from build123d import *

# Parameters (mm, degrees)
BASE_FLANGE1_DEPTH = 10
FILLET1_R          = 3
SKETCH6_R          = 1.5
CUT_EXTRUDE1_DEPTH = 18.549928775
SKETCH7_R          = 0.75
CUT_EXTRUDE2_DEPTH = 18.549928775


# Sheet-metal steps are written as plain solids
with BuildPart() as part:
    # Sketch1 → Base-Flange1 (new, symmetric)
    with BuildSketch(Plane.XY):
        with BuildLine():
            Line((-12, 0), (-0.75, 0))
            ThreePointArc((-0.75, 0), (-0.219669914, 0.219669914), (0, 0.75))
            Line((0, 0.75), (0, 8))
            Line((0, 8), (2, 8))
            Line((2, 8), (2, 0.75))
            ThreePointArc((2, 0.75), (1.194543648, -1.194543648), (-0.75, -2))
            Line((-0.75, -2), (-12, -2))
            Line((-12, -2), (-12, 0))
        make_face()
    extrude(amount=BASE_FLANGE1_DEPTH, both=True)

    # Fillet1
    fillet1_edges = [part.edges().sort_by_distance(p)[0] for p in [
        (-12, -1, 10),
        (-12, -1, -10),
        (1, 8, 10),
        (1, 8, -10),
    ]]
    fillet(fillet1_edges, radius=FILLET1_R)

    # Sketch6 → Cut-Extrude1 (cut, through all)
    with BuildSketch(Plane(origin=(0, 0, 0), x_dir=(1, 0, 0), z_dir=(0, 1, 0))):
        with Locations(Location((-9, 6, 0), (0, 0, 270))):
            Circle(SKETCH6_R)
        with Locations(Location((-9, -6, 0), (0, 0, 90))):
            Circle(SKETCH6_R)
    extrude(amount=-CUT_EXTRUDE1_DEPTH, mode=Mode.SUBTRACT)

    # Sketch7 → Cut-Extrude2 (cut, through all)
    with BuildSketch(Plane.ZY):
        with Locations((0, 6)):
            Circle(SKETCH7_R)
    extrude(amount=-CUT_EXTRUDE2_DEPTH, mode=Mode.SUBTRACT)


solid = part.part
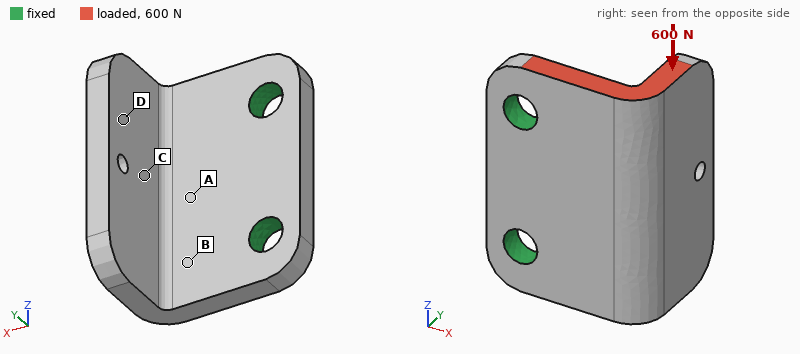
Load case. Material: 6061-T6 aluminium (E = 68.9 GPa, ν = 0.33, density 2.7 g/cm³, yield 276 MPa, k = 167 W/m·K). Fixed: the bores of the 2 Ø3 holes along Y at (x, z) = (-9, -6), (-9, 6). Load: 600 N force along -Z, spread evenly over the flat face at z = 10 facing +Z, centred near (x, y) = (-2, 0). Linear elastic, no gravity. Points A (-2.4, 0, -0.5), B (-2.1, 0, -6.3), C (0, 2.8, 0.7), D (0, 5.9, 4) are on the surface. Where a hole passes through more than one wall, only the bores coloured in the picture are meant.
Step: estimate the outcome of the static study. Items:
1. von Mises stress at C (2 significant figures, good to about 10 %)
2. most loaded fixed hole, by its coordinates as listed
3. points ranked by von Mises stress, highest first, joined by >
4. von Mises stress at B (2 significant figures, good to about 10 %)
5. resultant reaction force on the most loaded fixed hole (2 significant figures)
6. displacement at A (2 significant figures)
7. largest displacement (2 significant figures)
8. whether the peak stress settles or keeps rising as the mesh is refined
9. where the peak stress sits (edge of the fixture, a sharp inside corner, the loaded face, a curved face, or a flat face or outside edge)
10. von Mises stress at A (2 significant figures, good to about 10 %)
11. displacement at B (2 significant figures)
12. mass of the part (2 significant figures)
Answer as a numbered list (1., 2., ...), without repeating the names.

1. 16 MPa
2. (-9, 6)
3. A > B > C > D
4. 34 MPa
5. 450 N
6. 4.9 µm
7. 28 µm
8. keeps rising
9. edge of the fixture
10. 46 MPa
11. 8.6 µm
12. 2.2 g
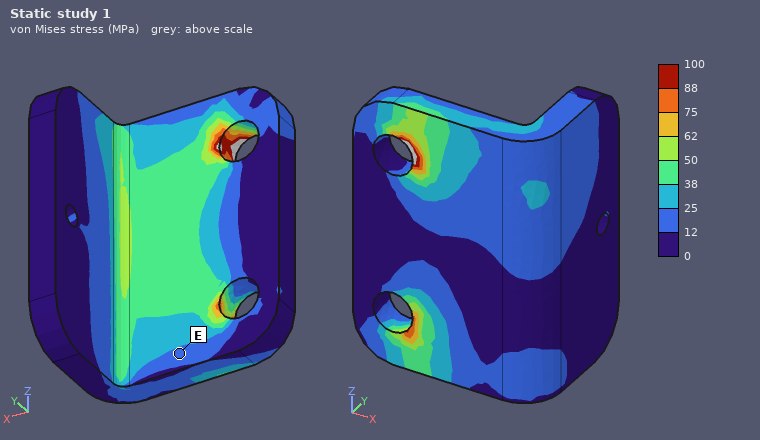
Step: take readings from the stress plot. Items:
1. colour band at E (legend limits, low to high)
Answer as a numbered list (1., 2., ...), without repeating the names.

1. 12 to 25 MPa
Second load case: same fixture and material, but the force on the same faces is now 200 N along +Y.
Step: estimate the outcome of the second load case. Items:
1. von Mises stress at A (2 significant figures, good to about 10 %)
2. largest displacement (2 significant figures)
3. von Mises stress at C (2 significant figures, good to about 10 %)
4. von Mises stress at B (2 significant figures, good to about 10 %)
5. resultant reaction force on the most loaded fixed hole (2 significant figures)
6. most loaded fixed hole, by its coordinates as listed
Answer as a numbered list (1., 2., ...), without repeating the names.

1. 45 MPa
2. 93 µm
3. 21 MPa
4. 41 MPa
5. 230 N
6. (-9, 6)
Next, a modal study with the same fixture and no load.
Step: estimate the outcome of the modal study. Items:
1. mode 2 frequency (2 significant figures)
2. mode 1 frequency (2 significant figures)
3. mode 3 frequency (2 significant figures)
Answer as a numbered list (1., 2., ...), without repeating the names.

1. 12 kHz
2. 6900 Hz
3. 19 kHz
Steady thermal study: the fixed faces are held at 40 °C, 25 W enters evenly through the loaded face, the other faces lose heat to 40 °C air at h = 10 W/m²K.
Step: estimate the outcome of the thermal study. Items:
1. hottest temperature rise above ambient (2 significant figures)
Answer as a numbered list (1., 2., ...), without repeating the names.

1. 51 K
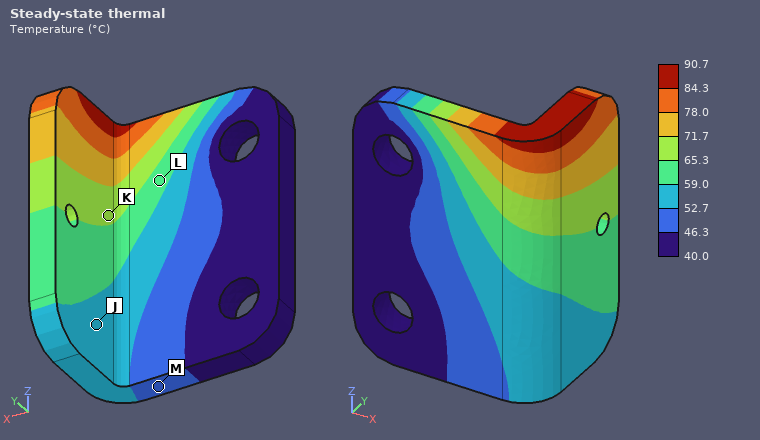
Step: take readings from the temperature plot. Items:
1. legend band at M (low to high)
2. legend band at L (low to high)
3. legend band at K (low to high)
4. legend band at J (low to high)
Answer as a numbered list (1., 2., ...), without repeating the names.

1. 46.3 to 52.7 °C
2. 59.0 to 65.3 °C
3. 65.3 to 71.7 °C
4. 52.7 to 59.0 °C
